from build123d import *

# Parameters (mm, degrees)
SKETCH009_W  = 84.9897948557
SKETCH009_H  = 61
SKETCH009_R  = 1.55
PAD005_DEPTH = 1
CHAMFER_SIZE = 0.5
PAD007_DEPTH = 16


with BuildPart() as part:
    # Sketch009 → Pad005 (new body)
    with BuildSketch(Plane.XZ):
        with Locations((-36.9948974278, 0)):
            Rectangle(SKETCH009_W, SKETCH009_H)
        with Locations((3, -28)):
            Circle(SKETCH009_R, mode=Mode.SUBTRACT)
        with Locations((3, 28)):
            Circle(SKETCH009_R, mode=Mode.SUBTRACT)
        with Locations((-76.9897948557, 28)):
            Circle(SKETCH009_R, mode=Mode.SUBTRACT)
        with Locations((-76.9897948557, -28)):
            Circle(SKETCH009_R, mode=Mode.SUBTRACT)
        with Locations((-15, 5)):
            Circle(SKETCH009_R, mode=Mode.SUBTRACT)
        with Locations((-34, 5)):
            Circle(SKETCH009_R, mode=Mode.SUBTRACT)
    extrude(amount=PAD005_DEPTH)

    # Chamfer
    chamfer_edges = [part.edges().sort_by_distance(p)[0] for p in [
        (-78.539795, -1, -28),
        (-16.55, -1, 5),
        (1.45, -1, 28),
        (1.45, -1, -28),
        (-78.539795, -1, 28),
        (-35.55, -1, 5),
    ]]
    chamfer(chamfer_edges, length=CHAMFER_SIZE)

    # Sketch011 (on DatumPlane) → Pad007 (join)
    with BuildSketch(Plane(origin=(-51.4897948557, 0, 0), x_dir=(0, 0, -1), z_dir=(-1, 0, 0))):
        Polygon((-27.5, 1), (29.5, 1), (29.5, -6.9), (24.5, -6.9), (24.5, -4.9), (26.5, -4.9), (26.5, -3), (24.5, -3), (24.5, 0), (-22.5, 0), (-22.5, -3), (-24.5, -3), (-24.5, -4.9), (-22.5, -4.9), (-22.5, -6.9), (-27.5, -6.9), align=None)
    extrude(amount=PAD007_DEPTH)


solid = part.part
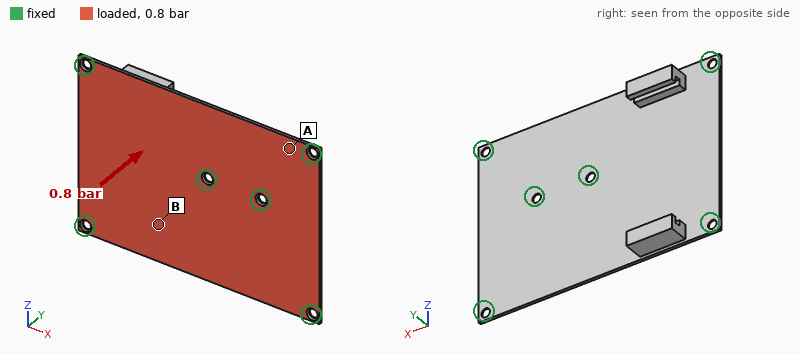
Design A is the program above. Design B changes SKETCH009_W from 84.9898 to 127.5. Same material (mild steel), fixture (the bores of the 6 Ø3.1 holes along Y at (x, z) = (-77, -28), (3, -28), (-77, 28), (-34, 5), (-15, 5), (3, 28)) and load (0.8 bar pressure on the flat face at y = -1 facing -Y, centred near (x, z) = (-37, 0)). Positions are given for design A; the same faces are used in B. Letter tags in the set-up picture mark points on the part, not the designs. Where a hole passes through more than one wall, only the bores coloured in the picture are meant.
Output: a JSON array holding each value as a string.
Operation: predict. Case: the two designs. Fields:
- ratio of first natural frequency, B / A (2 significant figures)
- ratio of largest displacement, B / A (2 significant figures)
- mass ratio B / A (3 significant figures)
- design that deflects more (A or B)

["0.85", "1.7", "1.42", "B"]
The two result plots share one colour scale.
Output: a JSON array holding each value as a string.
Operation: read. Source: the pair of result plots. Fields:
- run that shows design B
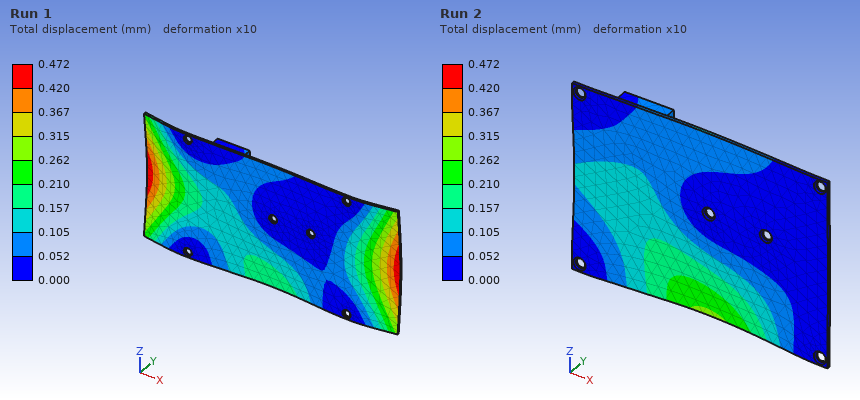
["Run 1"]
